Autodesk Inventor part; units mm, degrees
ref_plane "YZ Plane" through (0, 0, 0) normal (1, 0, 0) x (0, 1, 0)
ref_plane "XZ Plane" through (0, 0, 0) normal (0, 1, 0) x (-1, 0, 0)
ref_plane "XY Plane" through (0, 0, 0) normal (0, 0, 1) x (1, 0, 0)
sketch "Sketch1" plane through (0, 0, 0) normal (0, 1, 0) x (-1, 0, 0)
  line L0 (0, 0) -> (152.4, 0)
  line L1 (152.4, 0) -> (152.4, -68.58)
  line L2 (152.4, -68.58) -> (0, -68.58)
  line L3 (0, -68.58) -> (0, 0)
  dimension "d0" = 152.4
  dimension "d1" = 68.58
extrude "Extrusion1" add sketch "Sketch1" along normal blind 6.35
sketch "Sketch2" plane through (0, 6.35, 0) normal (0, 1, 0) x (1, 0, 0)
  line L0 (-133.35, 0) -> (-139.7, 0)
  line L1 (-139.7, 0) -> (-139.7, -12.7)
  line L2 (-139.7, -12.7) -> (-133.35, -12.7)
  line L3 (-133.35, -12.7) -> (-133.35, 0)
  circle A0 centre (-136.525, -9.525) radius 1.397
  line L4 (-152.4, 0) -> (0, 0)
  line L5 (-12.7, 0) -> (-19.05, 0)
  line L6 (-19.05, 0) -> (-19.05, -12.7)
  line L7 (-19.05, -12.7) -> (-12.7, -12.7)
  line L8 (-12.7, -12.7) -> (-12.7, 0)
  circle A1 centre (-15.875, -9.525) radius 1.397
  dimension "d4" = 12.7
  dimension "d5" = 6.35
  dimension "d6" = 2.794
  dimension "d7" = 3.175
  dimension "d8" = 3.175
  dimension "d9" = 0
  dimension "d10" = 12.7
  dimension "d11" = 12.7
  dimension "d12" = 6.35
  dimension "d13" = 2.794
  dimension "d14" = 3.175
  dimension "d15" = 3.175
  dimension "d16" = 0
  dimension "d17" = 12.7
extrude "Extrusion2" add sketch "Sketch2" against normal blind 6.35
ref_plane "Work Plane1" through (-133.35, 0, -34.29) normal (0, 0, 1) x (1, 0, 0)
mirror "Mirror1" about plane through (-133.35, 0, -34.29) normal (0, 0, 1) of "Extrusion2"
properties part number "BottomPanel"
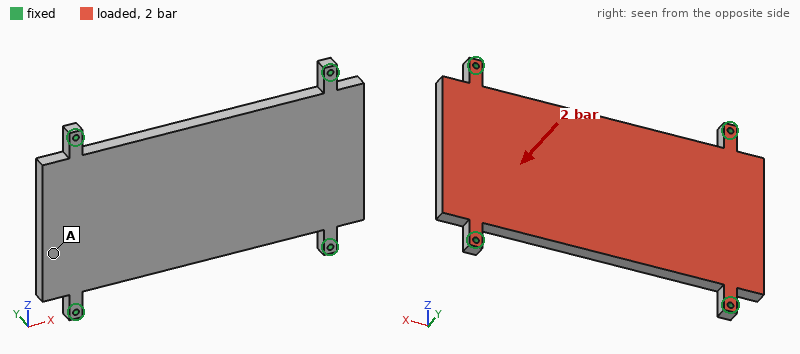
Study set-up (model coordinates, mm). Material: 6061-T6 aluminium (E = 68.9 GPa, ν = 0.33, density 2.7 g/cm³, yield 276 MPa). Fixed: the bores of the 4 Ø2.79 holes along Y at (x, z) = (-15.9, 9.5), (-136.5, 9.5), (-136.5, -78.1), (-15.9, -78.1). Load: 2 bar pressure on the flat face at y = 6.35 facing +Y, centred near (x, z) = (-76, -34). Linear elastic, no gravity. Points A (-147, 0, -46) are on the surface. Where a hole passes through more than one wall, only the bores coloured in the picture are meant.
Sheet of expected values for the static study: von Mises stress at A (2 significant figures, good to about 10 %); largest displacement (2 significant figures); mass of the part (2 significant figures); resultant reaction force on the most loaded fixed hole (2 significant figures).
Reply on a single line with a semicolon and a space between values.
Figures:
19 MPa; 0.28 mm; 180 g; 540 N
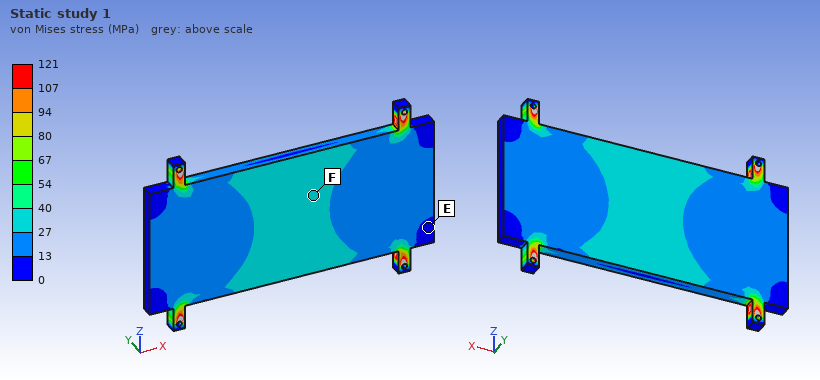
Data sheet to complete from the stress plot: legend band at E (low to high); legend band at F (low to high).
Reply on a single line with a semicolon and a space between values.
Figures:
0 to 13 MPa; 27 to 40 MPa
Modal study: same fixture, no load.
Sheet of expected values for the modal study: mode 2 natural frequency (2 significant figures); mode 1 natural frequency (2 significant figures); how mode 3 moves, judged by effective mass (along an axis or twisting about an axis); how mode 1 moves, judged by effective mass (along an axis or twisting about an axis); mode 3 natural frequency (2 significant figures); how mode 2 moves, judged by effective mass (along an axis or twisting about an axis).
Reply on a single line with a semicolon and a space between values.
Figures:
2700 Hz; 1100 Hz; twisting about Z; along Y; 2800 Hz; twisting about X
